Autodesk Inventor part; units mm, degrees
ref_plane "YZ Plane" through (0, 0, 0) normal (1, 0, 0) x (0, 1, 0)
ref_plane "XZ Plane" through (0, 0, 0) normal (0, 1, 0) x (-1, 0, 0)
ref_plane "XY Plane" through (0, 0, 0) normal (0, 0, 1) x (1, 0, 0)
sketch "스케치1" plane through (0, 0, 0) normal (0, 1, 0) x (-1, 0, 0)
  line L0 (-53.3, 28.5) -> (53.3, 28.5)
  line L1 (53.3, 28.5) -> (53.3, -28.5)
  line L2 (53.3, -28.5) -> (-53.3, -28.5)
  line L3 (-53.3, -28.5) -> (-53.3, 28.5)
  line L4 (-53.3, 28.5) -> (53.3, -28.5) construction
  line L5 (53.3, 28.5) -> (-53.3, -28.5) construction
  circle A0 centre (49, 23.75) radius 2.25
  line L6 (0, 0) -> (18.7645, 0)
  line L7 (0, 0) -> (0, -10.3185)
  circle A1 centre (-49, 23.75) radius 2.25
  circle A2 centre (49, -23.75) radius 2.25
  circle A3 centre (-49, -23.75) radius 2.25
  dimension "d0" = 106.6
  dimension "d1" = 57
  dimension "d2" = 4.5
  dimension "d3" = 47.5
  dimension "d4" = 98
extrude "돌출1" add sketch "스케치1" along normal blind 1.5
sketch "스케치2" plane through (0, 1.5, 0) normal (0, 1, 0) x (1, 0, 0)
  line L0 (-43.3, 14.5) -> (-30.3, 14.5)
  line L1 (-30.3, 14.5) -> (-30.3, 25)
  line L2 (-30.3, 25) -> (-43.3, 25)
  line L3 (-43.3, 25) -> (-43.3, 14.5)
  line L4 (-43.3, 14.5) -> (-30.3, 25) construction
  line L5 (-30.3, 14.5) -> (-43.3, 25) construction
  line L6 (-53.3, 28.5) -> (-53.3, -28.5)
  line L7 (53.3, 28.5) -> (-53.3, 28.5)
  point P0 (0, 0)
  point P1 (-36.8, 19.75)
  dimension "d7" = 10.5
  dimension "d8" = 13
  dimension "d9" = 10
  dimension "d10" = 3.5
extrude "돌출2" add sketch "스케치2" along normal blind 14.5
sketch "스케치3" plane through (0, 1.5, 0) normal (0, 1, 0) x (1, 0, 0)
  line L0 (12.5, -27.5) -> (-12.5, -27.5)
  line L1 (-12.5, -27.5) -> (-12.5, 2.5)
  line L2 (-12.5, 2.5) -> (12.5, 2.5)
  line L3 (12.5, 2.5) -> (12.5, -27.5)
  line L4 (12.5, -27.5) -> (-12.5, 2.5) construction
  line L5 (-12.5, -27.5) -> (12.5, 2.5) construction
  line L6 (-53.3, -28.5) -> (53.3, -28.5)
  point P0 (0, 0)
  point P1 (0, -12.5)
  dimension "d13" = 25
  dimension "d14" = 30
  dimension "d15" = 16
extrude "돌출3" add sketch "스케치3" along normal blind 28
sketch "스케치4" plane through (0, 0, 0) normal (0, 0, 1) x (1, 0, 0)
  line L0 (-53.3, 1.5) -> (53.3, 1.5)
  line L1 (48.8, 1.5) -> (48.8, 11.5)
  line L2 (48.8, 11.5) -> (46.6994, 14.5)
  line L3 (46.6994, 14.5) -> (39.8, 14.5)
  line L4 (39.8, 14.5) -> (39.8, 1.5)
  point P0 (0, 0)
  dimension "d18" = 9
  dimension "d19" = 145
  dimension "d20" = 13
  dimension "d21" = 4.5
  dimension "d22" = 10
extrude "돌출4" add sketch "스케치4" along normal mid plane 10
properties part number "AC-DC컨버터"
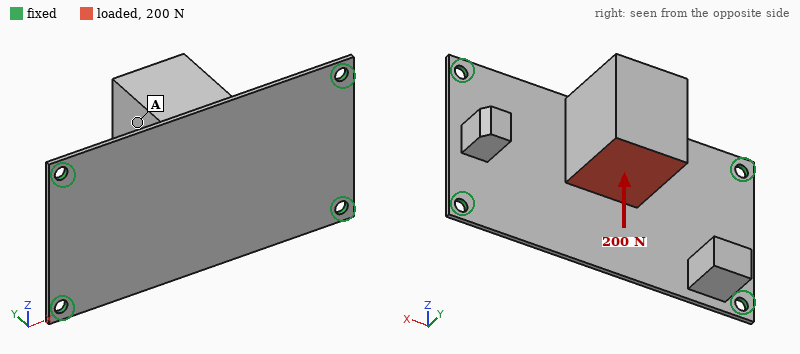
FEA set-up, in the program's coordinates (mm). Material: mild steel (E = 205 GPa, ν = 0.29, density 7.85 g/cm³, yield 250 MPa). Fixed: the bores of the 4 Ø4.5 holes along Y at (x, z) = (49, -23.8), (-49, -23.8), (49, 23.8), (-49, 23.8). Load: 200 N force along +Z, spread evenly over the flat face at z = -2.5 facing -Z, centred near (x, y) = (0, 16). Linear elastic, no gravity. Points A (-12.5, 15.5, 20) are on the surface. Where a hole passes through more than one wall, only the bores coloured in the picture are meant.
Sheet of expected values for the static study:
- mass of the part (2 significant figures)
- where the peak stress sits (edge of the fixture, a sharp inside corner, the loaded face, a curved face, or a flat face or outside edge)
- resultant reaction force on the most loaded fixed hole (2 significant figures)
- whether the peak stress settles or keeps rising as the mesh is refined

260 g
edge of the fixture
82 N
keeps rising
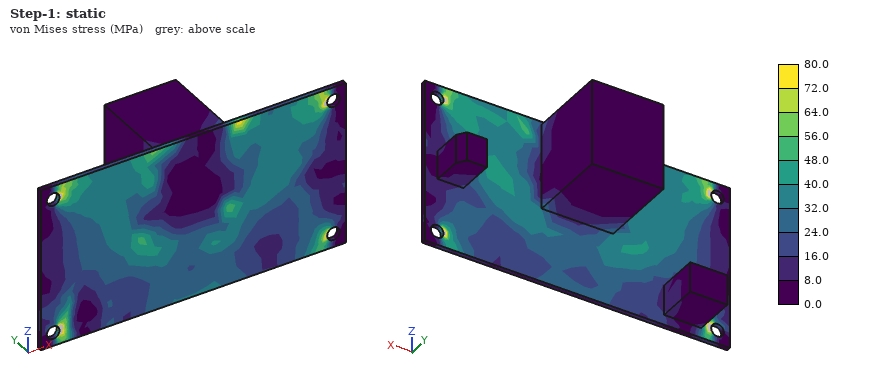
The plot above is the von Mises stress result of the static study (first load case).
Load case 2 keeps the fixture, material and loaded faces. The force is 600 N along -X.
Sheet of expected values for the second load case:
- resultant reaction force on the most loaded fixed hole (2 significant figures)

190 N
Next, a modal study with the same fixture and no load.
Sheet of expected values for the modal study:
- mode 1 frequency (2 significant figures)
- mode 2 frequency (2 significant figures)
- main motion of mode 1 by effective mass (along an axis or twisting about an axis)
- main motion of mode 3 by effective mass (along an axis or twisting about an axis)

380 Hz
520 Hz
along Y
along X
